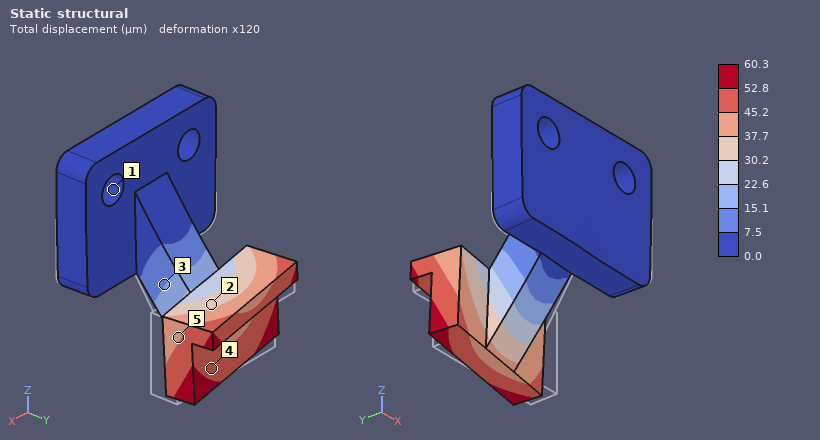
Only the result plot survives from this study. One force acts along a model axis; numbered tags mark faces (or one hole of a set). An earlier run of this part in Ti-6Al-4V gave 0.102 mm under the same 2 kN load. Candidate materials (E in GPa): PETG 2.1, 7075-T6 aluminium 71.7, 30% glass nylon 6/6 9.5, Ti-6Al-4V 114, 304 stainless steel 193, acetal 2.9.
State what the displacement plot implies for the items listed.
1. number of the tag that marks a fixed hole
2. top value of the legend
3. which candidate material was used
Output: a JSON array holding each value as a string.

["1", "60.3 µm", "304 stainless steel"]
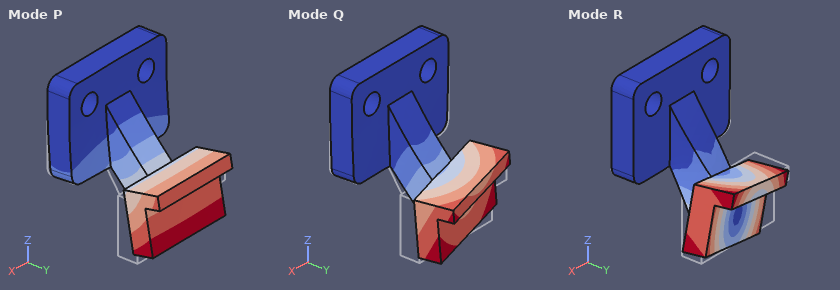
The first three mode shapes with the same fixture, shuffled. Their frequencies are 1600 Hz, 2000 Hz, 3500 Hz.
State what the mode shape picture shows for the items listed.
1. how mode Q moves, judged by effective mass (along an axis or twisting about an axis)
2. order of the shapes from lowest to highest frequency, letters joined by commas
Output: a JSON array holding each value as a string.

["along X", "P, Q, R"]
